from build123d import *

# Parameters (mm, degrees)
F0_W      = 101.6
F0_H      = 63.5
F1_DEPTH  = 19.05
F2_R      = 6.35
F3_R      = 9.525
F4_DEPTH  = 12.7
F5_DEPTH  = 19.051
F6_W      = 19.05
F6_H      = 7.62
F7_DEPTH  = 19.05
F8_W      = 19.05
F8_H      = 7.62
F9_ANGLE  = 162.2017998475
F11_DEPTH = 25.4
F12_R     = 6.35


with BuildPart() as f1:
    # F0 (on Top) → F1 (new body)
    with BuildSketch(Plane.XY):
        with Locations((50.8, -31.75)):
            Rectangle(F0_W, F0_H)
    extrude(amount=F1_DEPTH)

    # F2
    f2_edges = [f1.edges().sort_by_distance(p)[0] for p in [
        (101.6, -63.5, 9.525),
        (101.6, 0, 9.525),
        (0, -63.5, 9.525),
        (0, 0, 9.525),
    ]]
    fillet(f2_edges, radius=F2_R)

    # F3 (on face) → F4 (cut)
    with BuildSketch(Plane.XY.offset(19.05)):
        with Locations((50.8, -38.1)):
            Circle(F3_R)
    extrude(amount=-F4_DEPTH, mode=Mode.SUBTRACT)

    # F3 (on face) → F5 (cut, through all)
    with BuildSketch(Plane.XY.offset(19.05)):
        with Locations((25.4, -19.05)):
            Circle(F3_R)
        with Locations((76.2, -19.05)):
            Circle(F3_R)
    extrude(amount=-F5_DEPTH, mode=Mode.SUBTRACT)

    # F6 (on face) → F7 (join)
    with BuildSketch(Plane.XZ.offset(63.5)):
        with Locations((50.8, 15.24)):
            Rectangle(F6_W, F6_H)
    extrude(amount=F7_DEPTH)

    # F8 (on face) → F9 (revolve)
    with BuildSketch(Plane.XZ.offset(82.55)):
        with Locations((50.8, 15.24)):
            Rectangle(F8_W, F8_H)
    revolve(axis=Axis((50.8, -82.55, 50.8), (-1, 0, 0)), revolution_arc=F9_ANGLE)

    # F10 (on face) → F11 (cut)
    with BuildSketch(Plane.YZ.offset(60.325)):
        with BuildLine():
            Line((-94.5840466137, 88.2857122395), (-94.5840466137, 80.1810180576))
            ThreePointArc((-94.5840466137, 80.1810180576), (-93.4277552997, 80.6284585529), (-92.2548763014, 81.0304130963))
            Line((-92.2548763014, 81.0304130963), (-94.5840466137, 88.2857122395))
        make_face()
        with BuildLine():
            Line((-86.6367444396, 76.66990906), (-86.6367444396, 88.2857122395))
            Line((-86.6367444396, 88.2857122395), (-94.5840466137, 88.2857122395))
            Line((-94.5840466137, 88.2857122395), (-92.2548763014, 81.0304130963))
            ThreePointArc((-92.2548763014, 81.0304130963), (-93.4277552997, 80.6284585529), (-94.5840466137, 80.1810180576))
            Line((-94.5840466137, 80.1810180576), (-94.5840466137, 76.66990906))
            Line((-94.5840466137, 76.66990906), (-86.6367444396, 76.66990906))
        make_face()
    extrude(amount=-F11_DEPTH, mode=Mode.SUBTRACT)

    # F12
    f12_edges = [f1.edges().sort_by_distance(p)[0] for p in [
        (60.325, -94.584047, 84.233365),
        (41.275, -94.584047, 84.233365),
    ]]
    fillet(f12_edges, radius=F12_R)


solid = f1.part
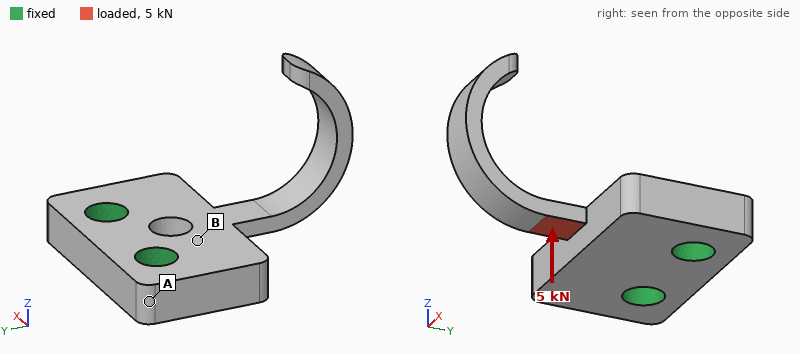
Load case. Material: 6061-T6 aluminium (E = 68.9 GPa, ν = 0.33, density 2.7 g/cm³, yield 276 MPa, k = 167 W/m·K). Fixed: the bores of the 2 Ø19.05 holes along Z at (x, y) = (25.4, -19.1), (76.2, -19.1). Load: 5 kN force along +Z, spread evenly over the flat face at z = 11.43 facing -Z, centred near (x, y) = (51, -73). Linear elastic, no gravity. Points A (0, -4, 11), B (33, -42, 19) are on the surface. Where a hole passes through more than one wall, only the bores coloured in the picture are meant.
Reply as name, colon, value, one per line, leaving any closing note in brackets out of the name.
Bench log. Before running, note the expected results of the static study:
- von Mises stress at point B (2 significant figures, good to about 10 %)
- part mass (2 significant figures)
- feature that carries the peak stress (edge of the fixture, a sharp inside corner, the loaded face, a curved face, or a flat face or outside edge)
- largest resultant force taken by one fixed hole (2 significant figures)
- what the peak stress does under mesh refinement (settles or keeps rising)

von Mises stress at point B: 39 MPa
part mass: 340 g
feature that carries the peak stress: a sharp inside corner
largest resultant force taken by one fixed hole: 2.5 kN
what the peak stress does under mesh refinement: keeps rising
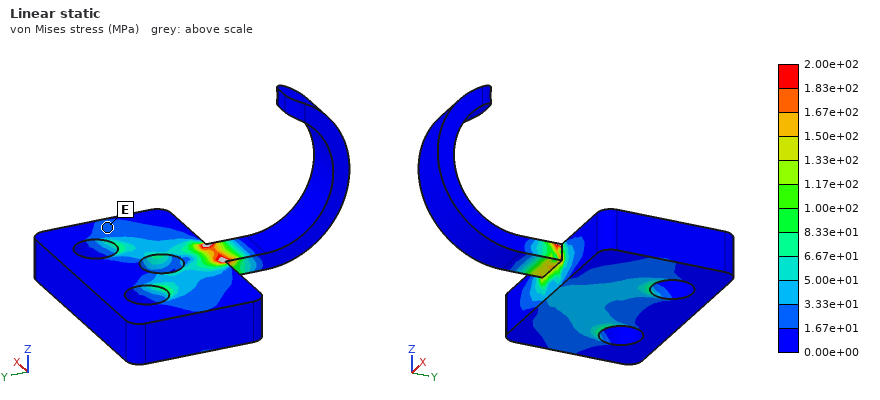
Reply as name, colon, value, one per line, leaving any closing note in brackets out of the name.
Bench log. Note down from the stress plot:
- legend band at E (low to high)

legend band at E: 1.67e+01 to 3.33e+01 MPa
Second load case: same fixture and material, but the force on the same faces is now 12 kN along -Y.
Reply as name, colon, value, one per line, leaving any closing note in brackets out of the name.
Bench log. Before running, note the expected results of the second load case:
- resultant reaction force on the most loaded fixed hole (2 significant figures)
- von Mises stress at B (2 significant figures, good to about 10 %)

resultant reaction force on the most loaded fixed hole: 6.6 kN
von Mises stress at B: 22 MPa
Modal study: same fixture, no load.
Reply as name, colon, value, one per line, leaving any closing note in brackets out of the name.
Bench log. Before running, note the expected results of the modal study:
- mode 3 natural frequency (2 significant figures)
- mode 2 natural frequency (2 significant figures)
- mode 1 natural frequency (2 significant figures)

mode 3 natural frequency: 1500 Hz
mode 2 natural frequency: 720 Hz
mode 1 natural frequency: 520 Hz
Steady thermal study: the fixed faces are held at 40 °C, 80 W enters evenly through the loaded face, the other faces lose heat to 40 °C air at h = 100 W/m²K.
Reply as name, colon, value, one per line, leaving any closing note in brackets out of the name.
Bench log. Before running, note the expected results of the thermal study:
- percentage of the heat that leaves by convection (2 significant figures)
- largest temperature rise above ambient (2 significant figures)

percentage of the heat that leaves by convection: 27 %
largest temperature rise above ambient: 46 K
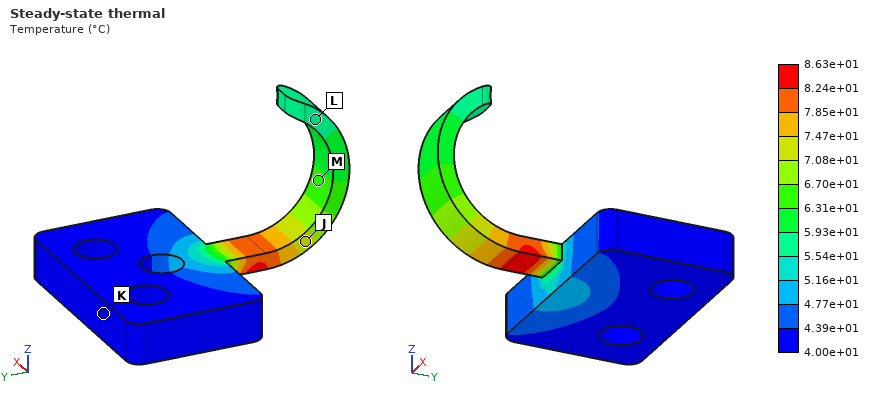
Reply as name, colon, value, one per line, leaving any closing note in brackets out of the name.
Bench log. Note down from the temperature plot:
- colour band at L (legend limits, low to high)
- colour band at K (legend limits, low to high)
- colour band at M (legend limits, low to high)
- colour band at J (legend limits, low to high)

colour band at L: 5.54e+01 to 5.93e+01 °C
colour band at K: 4.00e+01 to 4.39e+01 °C
colour band at M: 6.31e+01 to 6.70e+01 °C
colour band at J: 7.08e+01 to 7.47e+01 °C
